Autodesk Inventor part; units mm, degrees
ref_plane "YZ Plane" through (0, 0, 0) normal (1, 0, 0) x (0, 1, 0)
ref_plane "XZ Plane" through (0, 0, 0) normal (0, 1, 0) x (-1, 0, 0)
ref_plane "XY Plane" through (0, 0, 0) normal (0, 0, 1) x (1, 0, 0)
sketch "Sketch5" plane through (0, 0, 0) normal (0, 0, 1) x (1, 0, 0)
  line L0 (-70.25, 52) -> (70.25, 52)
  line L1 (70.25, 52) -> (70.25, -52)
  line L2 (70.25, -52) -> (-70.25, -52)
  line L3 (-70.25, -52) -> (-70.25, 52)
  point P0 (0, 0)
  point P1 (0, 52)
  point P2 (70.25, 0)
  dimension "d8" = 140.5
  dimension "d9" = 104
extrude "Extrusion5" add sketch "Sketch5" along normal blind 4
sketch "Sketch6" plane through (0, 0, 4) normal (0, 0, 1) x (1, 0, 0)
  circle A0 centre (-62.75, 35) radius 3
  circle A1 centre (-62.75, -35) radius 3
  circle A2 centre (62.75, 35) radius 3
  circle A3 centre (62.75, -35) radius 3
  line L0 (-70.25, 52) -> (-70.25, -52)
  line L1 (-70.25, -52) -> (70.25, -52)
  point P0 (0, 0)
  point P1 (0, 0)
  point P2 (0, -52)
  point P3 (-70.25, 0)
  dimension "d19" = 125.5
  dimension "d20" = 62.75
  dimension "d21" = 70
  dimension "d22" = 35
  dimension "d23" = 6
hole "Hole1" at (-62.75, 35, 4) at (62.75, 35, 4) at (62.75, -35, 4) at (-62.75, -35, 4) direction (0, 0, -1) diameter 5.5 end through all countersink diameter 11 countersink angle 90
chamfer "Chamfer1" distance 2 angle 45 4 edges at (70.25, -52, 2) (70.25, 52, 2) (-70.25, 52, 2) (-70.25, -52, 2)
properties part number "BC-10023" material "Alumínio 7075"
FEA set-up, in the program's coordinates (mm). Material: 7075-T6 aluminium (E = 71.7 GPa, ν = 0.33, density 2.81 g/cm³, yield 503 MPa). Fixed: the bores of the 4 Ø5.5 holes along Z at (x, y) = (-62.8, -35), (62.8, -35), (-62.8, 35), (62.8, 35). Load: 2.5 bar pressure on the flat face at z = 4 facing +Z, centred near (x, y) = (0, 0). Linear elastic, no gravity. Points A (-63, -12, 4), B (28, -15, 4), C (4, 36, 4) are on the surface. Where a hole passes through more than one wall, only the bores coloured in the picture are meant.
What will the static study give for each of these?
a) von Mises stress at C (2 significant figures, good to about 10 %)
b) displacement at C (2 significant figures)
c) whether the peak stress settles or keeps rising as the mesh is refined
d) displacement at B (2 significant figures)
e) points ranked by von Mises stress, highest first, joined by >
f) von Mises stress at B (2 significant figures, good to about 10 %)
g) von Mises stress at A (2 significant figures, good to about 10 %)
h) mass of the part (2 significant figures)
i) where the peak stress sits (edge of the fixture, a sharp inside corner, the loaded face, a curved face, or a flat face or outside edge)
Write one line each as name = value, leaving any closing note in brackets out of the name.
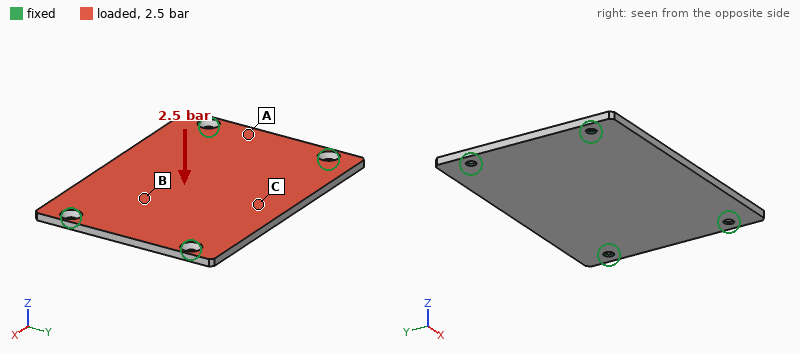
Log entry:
von Mises stress at C = 93 MPa
displacement at C = 0.74 mm
whether the peak stress settles or keeps rising as the mesh is refined = keeps rising
displacement at B = 0.56 mm
points ranked by von Mises stress, highest first, joined by > = C > B > A
von Mises stress at B = 55 MPa
von Mises stress at A = 29 MPa
mass of the part = 160 g
where the peak stress sits = edge of the fixture
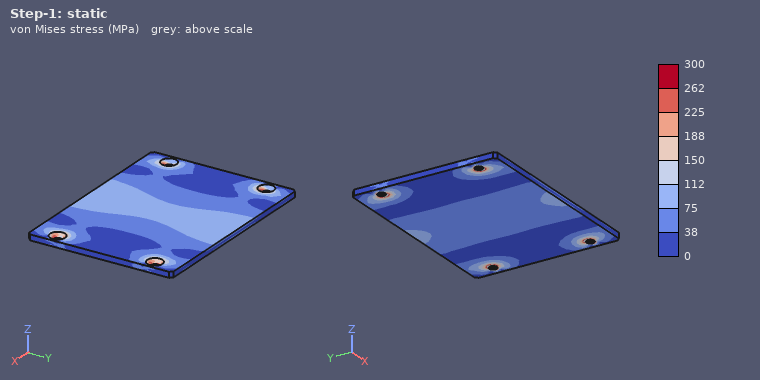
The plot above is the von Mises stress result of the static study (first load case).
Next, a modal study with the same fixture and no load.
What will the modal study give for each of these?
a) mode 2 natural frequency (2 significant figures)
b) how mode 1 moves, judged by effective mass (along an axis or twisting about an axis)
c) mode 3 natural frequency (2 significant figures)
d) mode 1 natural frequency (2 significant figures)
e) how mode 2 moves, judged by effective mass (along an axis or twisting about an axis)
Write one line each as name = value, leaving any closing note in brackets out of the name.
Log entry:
mode 2 natural frequency = 1400 Hz
how mode 1 moves, judged by effective mass = along Z
mode 3 natural frequency = 2500 Hz
mode 1 natural frequency = 980 Hz
how mode 2 moves, judged by effective mass = twisting about X
